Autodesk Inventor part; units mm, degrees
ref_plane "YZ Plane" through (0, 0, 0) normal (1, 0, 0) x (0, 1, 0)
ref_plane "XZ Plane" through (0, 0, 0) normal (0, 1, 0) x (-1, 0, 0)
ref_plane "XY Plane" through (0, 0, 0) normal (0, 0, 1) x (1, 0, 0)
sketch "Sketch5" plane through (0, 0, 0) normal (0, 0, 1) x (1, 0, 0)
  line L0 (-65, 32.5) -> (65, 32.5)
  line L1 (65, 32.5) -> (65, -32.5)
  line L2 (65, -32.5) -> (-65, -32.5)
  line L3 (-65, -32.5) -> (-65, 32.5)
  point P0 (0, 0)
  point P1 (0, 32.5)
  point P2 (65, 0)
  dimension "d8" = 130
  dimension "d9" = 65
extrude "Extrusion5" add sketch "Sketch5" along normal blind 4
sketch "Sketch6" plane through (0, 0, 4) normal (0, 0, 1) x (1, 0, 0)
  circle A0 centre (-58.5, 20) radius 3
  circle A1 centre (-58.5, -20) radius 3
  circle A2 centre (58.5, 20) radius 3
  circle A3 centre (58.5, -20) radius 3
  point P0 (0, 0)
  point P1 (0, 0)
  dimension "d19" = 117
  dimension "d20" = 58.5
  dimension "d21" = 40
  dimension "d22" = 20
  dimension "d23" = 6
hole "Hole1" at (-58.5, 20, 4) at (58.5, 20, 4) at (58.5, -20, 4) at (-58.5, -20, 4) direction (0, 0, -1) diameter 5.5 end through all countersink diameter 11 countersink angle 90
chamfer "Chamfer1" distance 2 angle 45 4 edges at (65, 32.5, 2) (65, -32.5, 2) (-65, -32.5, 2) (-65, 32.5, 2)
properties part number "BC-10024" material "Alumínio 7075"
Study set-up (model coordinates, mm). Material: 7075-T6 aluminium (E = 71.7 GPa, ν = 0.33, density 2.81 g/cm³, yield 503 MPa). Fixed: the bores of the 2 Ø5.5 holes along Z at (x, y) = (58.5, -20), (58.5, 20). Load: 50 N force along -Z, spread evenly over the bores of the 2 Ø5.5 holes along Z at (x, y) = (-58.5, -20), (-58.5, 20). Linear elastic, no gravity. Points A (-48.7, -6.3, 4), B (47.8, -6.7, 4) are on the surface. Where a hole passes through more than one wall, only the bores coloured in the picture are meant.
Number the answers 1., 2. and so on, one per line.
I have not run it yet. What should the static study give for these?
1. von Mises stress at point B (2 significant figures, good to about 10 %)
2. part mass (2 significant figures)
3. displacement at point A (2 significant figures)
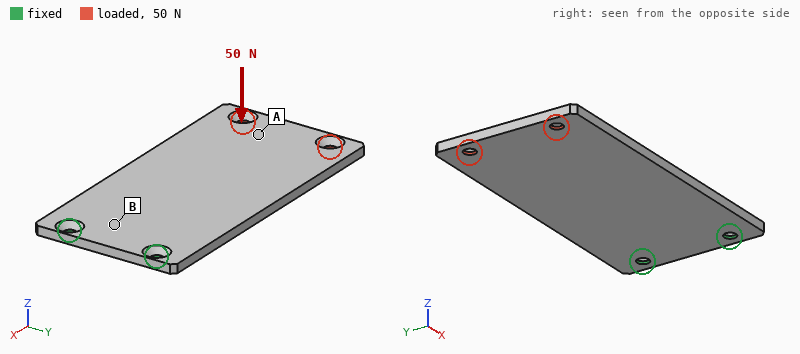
1. 28 MPa
2. 93 g
3. 1.2 mm
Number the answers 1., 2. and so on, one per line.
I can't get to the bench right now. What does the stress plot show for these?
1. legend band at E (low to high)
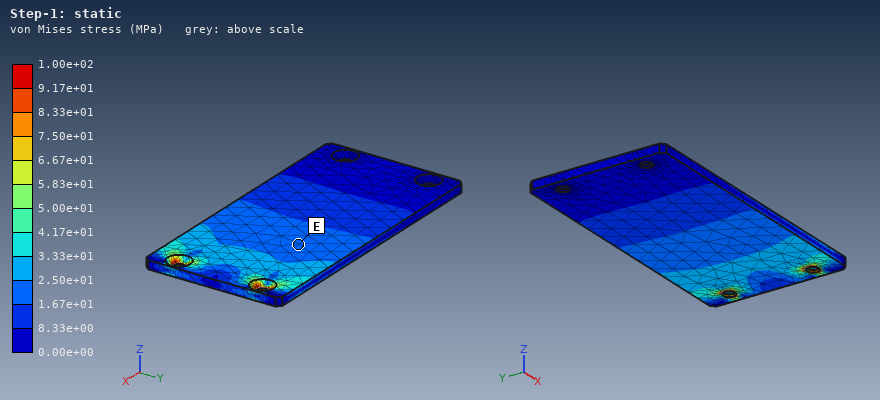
1. 1.67e+01 to 2.50e+01 MPa
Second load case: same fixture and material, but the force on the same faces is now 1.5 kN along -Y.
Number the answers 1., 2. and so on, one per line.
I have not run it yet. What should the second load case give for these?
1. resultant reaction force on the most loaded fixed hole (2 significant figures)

1. 4.2 kN
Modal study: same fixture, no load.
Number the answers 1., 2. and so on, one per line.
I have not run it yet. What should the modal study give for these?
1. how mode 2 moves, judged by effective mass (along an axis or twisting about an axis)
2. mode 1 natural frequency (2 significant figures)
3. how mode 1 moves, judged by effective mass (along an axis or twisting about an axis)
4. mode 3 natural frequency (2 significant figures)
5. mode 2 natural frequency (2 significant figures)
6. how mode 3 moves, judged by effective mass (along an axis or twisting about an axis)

1. twisting about X
2. 180 Hz
3. along Z
4. 1200 Hz
5. 840 Hz
6. along Z
